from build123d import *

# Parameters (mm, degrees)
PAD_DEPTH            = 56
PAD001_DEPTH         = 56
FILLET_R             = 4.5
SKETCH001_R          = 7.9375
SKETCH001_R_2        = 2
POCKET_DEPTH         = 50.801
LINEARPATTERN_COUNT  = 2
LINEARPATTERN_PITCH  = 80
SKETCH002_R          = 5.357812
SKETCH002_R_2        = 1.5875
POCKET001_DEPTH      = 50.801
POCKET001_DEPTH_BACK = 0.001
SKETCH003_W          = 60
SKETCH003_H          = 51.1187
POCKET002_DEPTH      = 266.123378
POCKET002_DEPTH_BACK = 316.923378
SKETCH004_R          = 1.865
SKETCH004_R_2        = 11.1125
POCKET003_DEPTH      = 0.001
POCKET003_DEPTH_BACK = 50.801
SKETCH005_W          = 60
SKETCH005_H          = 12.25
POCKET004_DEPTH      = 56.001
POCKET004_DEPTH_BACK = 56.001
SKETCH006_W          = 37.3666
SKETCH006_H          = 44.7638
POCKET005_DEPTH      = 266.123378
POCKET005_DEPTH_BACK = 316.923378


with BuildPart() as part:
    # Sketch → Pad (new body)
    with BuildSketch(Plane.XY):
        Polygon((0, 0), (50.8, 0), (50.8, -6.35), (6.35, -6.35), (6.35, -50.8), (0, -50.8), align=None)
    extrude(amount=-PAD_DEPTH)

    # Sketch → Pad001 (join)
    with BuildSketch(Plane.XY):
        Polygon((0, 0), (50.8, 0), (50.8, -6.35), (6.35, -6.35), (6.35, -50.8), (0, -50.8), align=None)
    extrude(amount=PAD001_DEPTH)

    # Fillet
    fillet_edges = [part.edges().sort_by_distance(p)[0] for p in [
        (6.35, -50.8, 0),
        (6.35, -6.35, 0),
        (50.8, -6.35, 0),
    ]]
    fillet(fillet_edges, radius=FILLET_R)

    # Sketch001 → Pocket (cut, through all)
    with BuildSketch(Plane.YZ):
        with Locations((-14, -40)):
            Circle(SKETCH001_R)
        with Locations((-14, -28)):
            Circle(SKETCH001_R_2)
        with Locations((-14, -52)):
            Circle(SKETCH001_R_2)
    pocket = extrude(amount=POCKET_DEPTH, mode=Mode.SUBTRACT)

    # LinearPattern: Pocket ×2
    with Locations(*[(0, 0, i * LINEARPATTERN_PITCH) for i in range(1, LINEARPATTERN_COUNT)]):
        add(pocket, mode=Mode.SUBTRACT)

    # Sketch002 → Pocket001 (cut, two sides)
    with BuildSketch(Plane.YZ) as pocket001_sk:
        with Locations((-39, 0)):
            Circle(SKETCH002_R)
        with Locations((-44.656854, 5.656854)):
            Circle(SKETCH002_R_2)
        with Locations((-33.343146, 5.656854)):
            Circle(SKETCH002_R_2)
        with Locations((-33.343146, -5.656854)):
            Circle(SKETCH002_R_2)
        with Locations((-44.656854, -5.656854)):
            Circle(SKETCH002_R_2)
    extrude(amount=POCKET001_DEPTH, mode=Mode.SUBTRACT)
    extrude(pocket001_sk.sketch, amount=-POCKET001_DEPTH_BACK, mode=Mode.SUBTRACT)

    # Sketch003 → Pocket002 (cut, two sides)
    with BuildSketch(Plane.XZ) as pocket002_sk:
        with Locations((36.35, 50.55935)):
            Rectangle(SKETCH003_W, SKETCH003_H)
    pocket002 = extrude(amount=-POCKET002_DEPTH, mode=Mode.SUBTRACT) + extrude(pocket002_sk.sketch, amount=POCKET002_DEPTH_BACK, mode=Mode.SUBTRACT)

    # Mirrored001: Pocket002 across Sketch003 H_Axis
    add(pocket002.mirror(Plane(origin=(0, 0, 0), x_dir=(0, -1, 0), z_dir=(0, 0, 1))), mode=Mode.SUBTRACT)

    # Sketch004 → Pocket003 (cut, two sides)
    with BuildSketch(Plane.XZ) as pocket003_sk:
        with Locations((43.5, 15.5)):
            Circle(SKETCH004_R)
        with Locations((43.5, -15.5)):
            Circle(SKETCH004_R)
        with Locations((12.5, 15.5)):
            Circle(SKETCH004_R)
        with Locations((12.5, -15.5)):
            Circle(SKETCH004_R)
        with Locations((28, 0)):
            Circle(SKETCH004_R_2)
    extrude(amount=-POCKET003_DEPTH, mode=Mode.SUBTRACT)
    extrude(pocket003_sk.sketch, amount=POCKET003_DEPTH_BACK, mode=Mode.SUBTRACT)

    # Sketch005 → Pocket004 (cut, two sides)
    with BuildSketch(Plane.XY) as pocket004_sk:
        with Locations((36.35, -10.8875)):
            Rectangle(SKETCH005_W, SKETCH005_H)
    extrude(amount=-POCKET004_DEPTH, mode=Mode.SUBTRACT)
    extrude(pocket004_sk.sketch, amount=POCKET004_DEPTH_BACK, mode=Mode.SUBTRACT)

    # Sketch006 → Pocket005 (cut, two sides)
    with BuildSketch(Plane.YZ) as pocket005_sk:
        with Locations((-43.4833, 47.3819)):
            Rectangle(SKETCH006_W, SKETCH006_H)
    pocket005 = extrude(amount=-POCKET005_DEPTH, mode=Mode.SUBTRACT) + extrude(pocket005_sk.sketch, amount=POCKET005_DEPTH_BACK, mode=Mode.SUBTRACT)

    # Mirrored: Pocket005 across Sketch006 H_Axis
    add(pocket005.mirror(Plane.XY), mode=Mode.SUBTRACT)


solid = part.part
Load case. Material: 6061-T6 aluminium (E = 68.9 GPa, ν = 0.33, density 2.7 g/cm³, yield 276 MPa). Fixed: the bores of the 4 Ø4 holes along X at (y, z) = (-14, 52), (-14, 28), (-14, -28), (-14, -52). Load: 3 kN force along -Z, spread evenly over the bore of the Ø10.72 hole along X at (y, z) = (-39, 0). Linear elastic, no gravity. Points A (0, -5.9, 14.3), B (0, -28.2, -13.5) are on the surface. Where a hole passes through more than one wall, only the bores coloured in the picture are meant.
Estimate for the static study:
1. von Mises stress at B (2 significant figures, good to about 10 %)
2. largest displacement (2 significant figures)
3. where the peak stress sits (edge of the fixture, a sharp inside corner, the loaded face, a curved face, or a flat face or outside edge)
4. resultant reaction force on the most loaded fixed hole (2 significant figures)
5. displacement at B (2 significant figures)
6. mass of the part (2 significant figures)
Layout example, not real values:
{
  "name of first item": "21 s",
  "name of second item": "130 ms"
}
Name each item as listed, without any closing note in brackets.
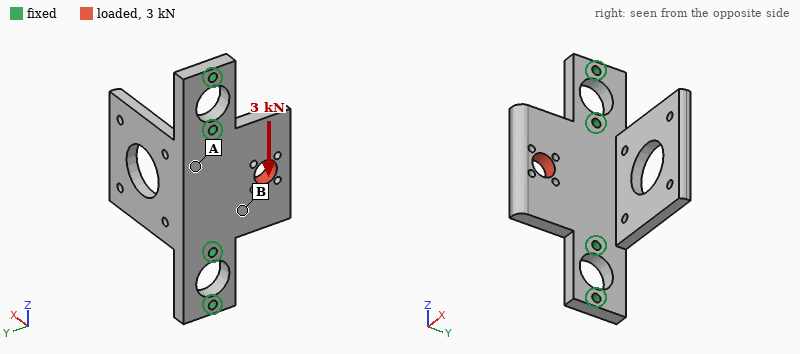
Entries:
{
  "von Mises stress at B": "16 MPa",
  "largest displacement": "21 µm",
  "where the peak stress sits": "a curved face",
  "resultant reaction force on the most loaded fixed hole": "1.9 kN",
  "displacement at B": "6.7 µm",
  "mass of the part": "82 g"
}
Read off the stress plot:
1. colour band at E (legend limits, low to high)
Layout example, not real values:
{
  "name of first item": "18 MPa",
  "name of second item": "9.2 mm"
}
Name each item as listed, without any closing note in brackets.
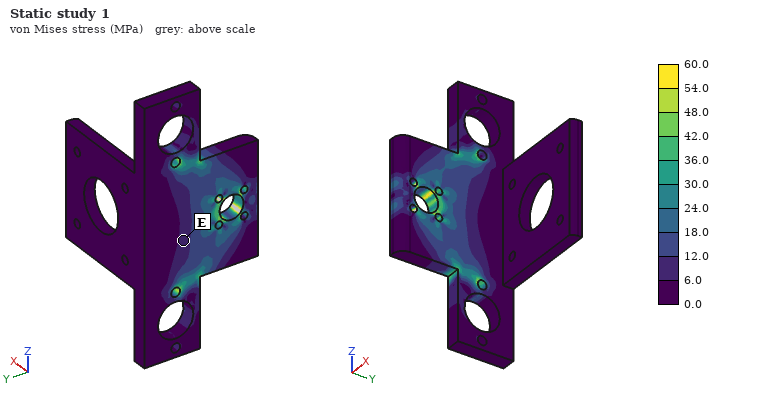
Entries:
{
  "colour band at E": "6.0 to 12.0 MPa"
}
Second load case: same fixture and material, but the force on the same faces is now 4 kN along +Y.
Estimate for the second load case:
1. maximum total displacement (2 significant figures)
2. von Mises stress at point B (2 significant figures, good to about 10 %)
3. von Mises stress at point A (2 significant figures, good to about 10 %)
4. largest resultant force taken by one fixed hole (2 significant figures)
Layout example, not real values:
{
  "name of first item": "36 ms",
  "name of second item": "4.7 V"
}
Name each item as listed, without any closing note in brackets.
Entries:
{
  "maximum total displacement": "21 µm",
  "von Mises stress at point B": "20 MPa",
  "von Mises stress at point A": "10 MPa",
  "largest resultant force taken by one fixed hole": "2.1 kN"
}
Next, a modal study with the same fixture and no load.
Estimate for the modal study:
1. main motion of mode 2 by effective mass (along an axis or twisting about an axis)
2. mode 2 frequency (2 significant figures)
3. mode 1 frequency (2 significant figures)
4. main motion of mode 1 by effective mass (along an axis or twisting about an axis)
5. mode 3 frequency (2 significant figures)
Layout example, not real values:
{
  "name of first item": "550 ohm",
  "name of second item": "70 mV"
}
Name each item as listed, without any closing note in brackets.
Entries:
{
  "main motion of mode 2 by effective mass": "along X",
  "mode 2 frequency": "3200 Hz",
  "mode 1 frequency": "1400 Hz",
  "main motion of mode 1 by effective mass": "along Y",
  "mode 3 frequency": "3400 Hz"
}
